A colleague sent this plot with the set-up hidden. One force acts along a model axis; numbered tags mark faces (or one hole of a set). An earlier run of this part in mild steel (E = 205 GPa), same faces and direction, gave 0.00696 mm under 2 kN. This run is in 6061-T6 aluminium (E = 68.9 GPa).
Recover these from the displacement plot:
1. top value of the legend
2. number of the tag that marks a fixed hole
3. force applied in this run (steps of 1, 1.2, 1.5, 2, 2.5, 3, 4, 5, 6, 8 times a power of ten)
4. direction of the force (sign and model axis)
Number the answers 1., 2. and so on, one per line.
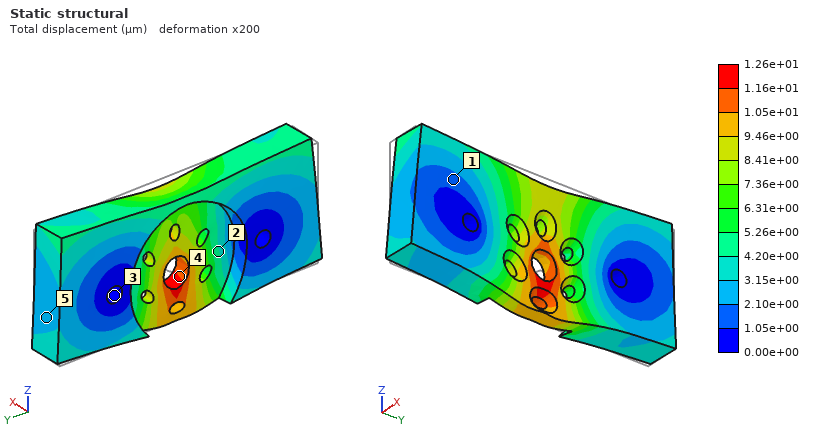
1. 1.26e+01 µm
2. 3
3. 1.2 kN
4. -Z
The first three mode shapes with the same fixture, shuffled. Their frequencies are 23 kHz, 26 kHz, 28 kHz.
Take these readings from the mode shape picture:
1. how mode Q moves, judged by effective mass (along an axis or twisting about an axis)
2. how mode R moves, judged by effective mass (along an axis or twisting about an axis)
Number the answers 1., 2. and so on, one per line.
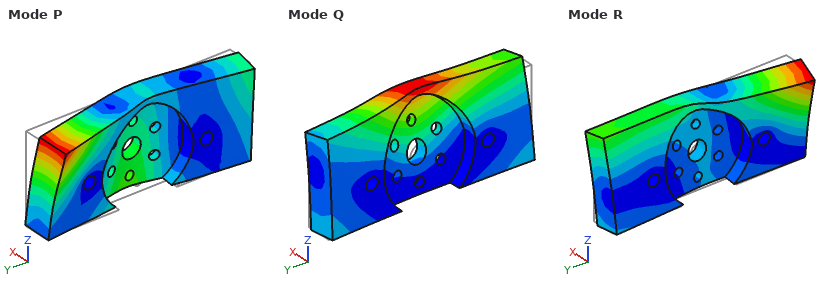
1. along X
2. twisting about Z
